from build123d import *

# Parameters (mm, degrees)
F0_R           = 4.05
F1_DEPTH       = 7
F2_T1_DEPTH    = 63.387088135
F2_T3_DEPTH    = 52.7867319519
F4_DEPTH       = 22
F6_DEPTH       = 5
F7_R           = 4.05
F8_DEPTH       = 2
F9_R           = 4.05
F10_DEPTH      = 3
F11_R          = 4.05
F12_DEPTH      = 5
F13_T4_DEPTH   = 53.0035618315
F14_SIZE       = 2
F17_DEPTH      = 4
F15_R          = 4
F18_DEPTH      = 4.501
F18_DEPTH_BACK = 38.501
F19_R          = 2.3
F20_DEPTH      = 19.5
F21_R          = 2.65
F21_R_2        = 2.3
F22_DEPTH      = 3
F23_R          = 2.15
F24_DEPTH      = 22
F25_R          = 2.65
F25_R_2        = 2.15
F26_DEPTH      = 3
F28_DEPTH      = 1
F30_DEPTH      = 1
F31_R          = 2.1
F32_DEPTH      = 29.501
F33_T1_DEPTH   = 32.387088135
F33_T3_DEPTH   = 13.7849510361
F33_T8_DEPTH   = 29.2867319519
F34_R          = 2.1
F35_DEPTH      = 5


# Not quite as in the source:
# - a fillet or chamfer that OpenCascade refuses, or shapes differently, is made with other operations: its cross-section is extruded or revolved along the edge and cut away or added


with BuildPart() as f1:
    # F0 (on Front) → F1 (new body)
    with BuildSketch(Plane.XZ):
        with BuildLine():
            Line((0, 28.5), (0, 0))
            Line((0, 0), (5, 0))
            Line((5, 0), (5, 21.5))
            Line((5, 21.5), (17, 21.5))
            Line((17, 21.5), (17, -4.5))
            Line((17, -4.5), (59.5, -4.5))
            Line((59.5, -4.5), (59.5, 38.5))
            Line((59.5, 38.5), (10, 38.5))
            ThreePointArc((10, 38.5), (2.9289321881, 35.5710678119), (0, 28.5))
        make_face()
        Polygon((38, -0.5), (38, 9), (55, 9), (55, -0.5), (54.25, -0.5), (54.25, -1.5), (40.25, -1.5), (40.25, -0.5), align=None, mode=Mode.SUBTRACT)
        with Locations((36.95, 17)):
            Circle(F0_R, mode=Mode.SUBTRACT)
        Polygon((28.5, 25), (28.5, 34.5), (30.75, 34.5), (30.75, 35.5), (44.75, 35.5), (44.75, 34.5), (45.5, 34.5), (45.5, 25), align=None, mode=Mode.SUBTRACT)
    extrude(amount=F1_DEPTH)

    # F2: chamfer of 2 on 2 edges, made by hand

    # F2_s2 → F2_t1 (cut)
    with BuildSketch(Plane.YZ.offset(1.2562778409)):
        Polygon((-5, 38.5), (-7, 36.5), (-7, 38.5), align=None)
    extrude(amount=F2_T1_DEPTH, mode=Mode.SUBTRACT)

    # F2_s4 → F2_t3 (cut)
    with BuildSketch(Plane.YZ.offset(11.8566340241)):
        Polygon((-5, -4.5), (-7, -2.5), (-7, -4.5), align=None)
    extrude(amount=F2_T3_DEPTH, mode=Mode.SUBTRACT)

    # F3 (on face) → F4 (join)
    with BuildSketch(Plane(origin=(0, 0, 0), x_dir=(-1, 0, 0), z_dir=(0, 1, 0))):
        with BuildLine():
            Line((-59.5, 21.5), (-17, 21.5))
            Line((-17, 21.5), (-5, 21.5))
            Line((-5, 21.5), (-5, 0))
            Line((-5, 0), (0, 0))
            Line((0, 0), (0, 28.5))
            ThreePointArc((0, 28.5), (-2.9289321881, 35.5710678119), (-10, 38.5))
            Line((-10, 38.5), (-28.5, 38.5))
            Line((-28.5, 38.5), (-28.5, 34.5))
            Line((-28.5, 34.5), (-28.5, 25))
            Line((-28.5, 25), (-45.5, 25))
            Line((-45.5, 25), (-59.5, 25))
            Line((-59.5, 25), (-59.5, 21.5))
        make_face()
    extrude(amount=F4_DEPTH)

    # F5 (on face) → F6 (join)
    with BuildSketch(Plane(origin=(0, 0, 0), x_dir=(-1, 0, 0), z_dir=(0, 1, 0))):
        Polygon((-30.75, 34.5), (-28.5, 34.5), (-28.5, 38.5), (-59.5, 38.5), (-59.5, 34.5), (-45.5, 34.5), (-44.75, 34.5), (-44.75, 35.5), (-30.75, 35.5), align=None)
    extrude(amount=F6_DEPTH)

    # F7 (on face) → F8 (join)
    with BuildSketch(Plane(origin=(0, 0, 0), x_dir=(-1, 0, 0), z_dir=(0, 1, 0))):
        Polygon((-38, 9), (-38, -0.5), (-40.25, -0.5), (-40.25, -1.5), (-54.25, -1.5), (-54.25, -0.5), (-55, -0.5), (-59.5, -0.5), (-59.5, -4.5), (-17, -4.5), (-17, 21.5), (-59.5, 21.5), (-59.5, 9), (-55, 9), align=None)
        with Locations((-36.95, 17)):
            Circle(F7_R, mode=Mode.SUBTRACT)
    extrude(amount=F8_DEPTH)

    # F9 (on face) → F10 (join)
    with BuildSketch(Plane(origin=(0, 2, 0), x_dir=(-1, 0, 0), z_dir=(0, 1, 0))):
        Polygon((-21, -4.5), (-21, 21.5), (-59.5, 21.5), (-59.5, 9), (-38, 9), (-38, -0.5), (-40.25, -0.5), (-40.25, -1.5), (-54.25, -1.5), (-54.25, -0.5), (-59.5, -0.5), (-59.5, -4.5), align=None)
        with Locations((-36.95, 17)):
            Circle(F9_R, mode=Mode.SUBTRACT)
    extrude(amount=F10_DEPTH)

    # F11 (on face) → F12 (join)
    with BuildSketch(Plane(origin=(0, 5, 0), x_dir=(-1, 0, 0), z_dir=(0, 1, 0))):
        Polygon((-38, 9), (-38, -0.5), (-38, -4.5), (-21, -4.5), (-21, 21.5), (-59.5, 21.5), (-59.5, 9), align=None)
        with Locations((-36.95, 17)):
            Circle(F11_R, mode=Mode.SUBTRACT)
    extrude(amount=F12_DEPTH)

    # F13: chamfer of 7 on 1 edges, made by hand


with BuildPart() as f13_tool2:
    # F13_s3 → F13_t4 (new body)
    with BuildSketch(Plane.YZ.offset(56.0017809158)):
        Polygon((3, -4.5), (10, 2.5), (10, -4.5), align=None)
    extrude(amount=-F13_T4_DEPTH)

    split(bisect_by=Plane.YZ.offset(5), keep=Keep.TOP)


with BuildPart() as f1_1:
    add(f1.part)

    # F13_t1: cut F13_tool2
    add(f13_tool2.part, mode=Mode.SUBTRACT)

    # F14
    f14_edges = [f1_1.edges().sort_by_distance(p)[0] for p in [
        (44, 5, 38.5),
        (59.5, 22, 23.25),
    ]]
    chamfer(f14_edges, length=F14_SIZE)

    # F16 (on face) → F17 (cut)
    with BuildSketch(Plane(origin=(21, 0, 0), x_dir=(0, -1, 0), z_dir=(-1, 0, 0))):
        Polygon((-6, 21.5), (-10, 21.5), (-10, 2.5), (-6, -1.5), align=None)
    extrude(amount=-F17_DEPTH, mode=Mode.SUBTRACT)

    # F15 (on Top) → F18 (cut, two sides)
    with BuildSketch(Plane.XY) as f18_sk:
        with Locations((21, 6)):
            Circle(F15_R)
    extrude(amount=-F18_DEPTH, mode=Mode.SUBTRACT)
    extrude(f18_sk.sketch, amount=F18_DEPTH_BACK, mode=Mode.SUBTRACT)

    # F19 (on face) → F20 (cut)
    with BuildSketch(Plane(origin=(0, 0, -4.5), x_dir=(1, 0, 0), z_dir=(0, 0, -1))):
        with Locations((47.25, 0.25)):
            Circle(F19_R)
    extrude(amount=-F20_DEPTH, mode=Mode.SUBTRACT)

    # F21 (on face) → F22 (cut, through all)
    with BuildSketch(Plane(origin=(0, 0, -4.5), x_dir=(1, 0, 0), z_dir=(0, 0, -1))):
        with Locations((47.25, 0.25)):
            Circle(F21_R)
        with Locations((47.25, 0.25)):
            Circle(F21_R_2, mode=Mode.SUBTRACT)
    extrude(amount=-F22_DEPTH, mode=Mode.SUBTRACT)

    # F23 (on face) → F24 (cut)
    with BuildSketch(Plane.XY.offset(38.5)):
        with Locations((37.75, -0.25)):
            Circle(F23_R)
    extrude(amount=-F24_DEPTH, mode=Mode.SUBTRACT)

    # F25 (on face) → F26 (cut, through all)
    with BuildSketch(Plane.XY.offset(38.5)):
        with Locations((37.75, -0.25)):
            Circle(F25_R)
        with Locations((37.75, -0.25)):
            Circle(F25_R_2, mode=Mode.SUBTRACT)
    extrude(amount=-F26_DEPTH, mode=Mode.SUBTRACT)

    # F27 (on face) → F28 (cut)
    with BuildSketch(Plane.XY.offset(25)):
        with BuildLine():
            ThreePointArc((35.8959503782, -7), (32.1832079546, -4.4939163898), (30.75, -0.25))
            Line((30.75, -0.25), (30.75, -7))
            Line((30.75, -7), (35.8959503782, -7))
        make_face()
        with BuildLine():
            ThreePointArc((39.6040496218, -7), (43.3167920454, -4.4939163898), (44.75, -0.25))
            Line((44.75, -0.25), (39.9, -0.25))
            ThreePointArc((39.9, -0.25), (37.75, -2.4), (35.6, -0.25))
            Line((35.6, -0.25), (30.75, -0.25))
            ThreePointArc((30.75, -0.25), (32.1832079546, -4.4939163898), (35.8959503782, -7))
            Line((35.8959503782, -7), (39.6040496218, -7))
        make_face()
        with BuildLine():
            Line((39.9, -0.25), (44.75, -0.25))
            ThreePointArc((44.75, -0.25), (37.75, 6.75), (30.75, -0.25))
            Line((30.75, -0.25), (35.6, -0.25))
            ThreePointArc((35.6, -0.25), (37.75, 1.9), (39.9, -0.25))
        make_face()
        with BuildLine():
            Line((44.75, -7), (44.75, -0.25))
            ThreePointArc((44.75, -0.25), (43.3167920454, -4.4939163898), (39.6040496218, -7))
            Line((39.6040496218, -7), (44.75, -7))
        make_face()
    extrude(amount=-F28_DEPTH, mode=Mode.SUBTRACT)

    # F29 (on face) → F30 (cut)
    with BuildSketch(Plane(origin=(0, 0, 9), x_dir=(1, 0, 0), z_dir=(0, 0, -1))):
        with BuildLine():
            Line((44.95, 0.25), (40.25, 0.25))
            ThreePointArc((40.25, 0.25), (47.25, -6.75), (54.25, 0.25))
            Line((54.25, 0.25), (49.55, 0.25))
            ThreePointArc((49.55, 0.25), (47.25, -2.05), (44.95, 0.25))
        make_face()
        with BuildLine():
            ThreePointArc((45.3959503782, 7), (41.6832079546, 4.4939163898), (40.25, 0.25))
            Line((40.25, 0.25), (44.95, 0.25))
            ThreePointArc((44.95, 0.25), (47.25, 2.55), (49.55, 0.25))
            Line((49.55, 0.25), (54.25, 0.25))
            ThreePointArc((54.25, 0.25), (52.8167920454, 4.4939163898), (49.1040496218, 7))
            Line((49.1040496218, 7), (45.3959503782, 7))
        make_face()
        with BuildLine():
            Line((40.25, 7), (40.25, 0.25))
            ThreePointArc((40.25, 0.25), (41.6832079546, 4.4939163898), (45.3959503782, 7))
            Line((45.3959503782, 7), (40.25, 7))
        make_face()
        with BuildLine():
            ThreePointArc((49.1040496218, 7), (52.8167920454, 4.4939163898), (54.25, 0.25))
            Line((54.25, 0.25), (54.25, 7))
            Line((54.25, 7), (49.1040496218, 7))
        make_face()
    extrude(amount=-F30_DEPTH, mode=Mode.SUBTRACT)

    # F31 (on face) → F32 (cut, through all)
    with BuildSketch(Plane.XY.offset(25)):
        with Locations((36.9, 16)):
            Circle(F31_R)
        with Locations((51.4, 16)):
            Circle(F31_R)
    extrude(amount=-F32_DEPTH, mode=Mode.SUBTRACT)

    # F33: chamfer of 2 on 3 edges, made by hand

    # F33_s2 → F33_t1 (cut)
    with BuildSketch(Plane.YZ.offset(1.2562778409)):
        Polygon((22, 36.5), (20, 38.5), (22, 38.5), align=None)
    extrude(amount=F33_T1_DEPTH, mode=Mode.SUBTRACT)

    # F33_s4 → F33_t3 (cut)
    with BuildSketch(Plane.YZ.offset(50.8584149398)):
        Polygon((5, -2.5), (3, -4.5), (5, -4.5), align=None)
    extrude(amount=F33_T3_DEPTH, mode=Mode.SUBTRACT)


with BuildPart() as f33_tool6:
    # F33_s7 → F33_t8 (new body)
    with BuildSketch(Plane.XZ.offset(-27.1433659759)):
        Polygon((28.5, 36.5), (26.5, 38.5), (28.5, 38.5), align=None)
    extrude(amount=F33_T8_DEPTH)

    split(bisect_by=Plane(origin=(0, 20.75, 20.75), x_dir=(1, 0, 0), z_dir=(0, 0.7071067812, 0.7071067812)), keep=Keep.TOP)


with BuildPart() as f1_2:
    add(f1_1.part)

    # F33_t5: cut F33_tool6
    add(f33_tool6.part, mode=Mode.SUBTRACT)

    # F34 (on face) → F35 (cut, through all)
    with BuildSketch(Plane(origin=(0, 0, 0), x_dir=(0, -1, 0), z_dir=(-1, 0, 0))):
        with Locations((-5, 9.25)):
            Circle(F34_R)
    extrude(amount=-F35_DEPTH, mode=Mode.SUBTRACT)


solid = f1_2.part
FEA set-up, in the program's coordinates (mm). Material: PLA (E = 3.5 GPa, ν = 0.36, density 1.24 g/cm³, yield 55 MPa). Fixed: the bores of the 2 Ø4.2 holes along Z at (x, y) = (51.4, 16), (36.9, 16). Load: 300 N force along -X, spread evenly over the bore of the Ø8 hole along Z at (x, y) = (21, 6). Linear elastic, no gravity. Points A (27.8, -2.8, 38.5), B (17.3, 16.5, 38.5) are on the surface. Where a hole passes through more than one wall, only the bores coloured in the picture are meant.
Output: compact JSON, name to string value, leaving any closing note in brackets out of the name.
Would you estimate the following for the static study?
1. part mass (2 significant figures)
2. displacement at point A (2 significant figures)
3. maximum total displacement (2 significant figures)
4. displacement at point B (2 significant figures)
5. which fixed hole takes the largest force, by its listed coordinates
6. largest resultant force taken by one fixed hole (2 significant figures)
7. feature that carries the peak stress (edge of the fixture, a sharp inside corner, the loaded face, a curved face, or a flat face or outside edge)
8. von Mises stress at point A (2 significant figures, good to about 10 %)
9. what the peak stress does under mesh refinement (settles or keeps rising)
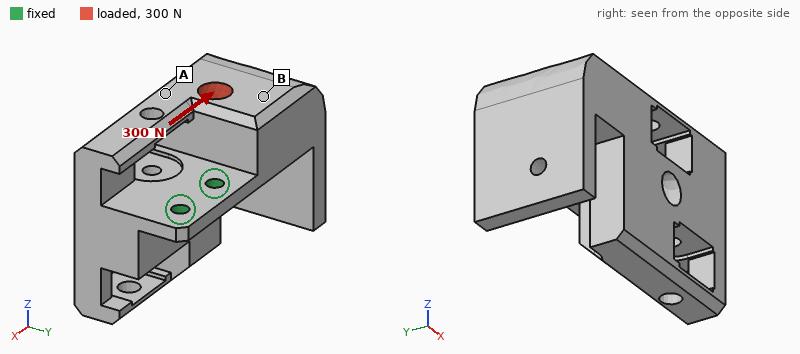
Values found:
{"part mass": "40 g", "displacement at point A": "0.13 mm", "maximum total displacement": "0.21 mm", "displacement at point B": "0.11 mm", "which fixed hole takes the largest force, by its listed coordinates": "(36.9, 16)", "largest resultant force taken by one fixed hole": "260 N", "feature that carries the peak stress": "edge of the fixture", "von Mises stress at point A": "3.0 MPa", "what the peak stress does under mesh refinement": "keeps rising"}
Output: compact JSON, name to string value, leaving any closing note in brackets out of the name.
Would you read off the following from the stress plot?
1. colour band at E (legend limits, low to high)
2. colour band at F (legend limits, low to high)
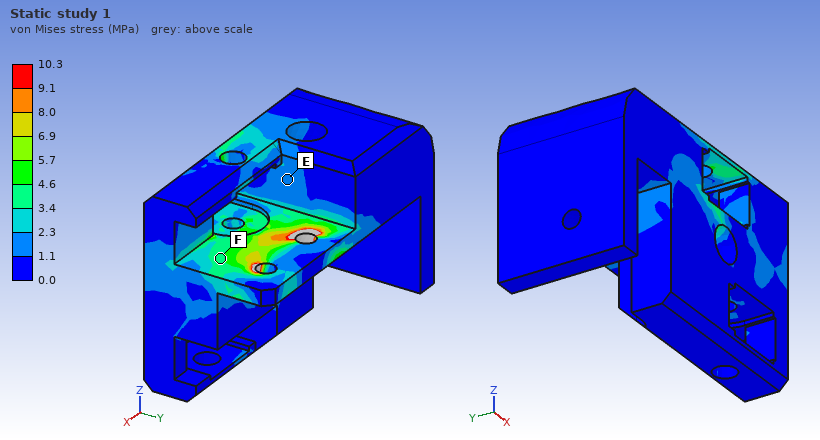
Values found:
{"colour band at E": "1.1 to 2.3 MPa", "colour band at F": "3.4 to 4.6 MPa"}
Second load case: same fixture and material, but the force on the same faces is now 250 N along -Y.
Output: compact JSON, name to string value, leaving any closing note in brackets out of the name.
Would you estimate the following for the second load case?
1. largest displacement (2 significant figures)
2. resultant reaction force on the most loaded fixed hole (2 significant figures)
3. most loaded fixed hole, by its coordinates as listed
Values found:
{"largest displacement": "0.25 mm", "resultant reaction force on the most loaded fixed hole": "440 N", "most loaded fixed hole, by its coordinates as listed": "(36.9, 16)"}
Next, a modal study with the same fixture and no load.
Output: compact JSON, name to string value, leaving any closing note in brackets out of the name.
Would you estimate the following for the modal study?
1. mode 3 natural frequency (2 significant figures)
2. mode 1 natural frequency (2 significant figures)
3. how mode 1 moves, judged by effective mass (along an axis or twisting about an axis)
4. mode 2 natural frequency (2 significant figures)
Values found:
{"mode 3 natural frequency": "1100 Hz", "mode 1 natural frequency": "410 Hz", "how mode 1 moves, judged by effective mass": "along Z", "mode 2 natural frequency": "690 Hz"}
